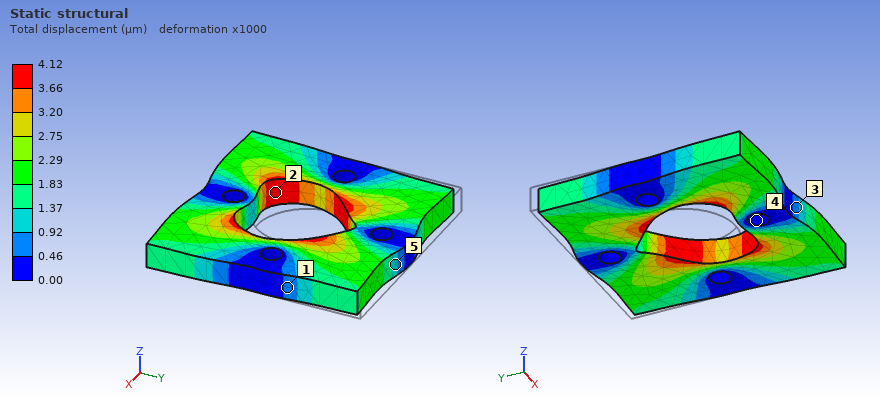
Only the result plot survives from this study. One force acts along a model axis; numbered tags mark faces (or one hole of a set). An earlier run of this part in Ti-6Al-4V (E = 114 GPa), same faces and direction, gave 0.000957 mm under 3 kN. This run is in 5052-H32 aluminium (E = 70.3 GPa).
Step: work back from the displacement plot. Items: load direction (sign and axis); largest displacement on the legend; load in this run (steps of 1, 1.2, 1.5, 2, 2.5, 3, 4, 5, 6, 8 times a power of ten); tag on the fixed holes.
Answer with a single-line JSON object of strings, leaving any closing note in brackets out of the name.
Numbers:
{"load direction": "-Y", "largest displacement on the legend": "4.12 µm", "load in this run": "8 kN", "tag on the fixed holes": "4"}
